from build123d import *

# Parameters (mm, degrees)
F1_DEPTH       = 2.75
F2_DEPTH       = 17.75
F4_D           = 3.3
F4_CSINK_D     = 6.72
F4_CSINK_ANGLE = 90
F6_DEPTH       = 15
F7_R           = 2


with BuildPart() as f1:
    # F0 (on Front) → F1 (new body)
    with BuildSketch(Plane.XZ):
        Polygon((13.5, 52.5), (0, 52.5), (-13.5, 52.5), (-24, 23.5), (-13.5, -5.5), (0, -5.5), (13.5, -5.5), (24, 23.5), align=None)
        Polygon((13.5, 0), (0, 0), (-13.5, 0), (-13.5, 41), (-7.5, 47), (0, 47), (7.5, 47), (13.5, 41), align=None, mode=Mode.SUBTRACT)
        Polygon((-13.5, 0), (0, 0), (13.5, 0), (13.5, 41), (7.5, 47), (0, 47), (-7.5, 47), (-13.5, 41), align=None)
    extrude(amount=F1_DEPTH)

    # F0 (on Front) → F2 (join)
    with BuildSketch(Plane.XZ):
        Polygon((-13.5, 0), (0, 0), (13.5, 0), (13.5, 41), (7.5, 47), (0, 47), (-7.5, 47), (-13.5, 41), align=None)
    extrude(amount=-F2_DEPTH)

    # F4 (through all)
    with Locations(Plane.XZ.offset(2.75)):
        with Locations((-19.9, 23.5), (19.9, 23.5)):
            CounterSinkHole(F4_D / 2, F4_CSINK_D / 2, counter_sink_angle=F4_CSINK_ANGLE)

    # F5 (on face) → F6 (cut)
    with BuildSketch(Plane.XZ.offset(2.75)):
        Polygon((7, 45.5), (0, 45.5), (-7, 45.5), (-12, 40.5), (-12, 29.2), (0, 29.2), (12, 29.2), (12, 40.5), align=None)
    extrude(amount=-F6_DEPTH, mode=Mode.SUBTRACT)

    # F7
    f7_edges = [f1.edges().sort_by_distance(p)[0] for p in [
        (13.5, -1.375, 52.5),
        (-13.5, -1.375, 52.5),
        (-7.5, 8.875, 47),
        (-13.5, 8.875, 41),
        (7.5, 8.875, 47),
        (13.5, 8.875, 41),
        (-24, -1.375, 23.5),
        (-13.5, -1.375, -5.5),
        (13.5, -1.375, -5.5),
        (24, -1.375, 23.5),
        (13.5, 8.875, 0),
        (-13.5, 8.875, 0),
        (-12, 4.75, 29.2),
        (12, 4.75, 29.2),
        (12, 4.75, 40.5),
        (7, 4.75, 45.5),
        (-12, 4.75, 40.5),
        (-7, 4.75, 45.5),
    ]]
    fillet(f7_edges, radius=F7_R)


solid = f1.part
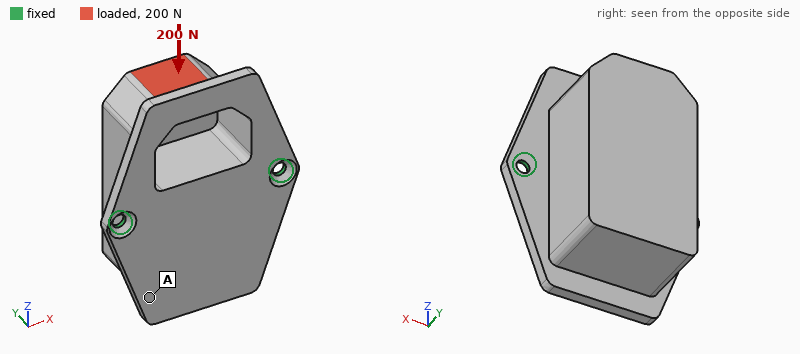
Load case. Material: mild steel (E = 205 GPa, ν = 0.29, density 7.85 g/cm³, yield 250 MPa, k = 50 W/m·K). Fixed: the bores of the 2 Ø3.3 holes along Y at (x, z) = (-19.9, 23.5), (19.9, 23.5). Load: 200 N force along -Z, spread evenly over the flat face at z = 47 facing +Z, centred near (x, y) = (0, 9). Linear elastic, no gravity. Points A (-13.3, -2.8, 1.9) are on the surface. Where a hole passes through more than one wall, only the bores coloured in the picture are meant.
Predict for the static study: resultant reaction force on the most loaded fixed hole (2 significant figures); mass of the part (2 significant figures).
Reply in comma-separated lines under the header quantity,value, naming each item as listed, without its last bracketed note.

quantity,value
resultant reaction force on the most loaded fixed hole,100 N
mass of the part,170 g
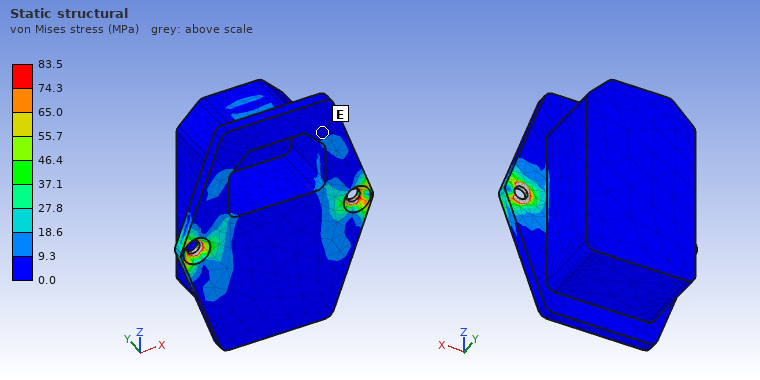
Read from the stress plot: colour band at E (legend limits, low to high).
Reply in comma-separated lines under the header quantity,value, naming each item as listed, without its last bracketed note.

quantity,value
colour band at E,0.0 to 9.3 MPa
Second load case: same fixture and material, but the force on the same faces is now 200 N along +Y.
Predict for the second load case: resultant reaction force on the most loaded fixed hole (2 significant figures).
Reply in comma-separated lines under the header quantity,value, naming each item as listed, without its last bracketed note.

quantity,value
resultant reaction force on the most loaded fixed hole,100 N
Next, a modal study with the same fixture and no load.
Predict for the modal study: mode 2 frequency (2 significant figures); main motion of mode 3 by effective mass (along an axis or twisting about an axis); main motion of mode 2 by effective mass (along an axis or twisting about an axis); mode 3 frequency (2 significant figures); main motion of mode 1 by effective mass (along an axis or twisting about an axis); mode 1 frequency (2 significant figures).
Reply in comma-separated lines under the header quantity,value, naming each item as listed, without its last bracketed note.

quantity,value
mode 2 frequency,4200 Hz
main motion of mode 3 by effective mass,along X
main motion of mode 2 by effective mass,along Y
mode 3 frequency,5000 Hz
main motion of mode 1 by effective mass,along Z
mode 1 frequency,870 Hz
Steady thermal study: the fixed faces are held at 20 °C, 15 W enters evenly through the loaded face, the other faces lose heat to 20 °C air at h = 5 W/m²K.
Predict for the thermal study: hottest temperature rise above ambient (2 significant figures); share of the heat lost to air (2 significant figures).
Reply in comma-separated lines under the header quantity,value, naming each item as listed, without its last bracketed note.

quantity,value
hottest temperature rise above ambient,76 K
share of the heat lost to air,9.9 %
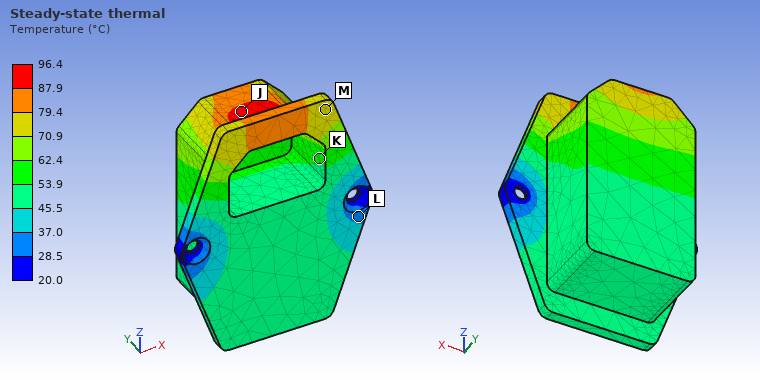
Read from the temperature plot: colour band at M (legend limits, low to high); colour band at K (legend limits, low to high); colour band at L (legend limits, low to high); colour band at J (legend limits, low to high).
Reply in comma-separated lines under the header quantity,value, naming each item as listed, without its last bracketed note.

quantity,value
colour band at M,70.9 to 79.4 °C
colour band at K,53.9 to 62.4 °C
colour band at L,28.5 to 37.0 °C
colour band at J,87.9 to 96.4 °C
